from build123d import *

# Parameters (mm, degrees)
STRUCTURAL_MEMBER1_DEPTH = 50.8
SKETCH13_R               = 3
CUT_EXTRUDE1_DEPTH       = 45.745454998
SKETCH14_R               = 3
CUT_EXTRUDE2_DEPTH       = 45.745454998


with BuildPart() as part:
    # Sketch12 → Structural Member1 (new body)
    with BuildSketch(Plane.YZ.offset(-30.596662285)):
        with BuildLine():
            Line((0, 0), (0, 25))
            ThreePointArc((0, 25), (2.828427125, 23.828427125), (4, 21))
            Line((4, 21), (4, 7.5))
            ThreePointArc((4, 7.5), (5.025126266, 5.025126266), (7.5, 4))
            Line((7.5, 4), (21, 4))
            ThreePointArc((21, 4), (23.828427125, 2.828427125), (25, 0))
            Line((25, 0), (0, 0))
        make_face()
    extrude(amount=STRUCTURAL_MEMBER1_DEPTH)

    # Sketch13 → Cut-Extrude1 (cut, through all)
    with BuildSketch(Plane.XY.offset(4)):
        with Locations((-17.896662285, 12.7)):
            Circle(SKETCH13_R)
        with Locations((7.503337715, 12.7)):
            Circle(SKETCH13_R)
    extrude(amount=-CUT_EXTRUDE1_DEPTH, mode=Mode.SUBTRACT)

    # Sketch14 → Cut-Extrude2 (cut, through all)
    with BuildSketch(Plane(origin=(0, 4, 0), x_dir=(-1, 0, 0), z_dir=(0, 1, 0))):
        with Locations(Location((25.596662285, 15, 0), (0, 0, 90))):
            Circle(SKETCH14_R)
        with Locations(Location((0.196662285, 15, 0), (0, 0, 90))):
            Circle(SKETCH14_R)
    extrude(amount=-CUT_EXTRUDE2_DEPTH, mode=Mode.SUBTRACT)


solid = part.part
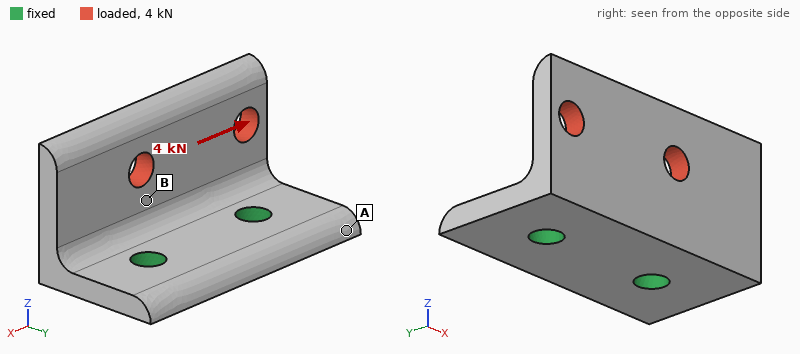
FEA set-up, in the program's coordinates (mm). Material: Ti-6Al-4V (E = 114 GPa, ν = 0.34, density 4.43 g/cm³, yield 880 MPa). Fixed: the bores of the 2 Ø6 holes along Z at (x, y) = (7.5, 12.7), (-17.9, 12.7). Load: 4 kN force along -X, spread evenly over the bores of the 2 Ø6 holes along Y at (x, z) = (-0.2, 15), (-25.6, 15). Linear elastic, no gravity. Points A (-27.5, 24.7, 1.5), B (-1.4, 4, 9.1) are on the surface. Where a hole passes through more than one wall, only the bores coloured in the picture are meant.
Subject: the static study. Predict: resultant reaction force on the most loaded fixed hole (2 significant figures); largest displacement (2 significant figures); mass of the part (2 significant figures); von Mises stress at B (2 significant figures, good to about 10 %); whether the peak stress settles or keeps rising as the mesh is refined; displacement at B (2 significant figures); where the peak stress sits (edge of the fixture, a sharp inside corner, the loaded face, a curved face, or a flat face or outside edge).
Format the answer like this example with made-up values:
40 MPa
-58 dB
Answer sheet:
3.0 kN
90 µm
38 g
110 MPa
keeps rising
22 µm
edge of the fixture
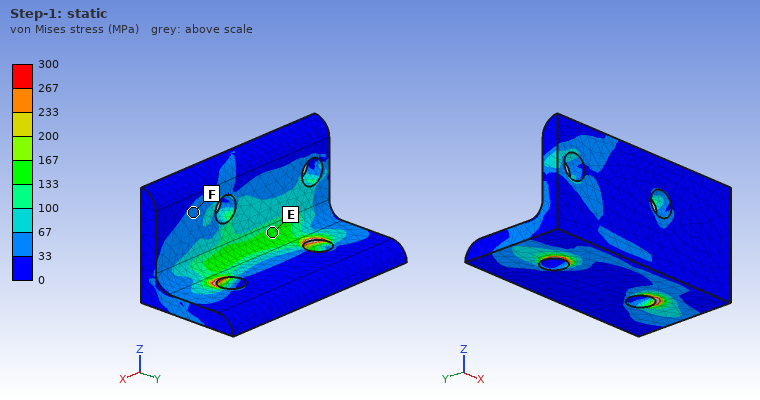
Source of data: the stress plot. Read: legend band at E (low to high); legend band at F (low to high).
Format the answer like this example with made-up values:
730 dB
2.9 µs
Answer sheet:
133 to 167 MPa
33 to 67 MPa
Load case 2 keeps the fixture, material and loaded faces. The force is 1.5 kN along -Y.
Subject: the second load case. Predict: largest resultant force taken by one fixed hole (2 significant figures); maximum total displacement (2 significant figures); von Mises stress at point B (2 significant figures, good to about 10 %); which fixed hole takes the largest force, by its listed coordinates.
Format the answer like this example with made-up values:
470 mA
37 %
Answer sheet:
1.1 kN
0.21 mm
61 MPa
(-17.9, 12.7)
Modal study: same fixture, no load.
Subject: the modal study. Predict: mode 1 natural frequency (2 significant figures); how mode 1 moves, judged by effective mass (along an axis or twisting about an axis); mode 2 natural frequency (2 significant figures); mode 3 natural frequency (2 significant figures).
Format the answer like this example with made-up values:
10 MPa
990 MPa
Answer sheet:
4500 Hz
along Y
6800 Hz
12 kHz
